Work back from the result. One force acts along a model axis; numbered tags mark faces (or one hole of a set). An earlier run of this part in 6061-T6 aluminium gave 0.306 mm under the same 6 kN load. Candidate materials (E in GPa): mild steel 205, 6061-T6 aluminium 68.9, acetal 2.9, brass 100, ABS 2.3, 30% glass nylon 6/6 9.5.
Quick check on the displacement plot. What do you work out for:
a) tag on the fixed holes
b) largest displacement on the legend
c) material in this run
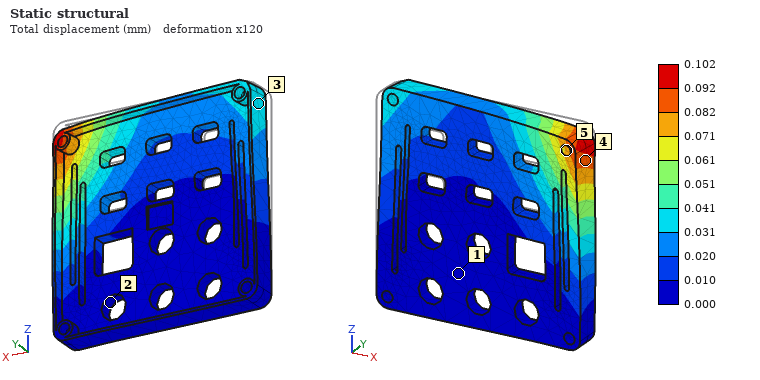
2
0.102 mm
mild steel
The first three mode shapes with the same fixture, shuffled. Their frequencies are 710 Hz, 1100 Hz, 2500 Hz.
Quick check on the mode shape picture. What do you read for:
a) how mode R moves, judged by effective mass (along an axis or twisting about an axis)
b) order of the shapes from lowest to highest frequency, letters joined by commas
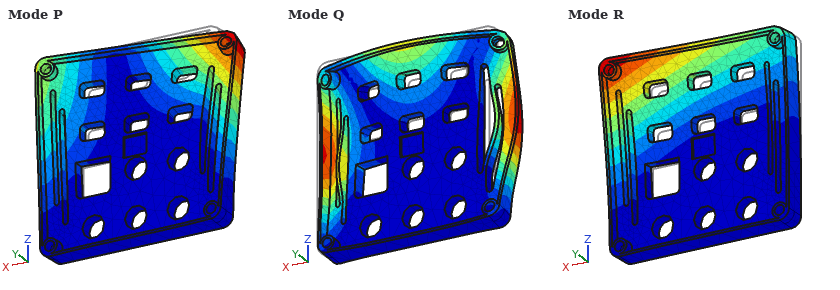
along Y
R, P, Q
